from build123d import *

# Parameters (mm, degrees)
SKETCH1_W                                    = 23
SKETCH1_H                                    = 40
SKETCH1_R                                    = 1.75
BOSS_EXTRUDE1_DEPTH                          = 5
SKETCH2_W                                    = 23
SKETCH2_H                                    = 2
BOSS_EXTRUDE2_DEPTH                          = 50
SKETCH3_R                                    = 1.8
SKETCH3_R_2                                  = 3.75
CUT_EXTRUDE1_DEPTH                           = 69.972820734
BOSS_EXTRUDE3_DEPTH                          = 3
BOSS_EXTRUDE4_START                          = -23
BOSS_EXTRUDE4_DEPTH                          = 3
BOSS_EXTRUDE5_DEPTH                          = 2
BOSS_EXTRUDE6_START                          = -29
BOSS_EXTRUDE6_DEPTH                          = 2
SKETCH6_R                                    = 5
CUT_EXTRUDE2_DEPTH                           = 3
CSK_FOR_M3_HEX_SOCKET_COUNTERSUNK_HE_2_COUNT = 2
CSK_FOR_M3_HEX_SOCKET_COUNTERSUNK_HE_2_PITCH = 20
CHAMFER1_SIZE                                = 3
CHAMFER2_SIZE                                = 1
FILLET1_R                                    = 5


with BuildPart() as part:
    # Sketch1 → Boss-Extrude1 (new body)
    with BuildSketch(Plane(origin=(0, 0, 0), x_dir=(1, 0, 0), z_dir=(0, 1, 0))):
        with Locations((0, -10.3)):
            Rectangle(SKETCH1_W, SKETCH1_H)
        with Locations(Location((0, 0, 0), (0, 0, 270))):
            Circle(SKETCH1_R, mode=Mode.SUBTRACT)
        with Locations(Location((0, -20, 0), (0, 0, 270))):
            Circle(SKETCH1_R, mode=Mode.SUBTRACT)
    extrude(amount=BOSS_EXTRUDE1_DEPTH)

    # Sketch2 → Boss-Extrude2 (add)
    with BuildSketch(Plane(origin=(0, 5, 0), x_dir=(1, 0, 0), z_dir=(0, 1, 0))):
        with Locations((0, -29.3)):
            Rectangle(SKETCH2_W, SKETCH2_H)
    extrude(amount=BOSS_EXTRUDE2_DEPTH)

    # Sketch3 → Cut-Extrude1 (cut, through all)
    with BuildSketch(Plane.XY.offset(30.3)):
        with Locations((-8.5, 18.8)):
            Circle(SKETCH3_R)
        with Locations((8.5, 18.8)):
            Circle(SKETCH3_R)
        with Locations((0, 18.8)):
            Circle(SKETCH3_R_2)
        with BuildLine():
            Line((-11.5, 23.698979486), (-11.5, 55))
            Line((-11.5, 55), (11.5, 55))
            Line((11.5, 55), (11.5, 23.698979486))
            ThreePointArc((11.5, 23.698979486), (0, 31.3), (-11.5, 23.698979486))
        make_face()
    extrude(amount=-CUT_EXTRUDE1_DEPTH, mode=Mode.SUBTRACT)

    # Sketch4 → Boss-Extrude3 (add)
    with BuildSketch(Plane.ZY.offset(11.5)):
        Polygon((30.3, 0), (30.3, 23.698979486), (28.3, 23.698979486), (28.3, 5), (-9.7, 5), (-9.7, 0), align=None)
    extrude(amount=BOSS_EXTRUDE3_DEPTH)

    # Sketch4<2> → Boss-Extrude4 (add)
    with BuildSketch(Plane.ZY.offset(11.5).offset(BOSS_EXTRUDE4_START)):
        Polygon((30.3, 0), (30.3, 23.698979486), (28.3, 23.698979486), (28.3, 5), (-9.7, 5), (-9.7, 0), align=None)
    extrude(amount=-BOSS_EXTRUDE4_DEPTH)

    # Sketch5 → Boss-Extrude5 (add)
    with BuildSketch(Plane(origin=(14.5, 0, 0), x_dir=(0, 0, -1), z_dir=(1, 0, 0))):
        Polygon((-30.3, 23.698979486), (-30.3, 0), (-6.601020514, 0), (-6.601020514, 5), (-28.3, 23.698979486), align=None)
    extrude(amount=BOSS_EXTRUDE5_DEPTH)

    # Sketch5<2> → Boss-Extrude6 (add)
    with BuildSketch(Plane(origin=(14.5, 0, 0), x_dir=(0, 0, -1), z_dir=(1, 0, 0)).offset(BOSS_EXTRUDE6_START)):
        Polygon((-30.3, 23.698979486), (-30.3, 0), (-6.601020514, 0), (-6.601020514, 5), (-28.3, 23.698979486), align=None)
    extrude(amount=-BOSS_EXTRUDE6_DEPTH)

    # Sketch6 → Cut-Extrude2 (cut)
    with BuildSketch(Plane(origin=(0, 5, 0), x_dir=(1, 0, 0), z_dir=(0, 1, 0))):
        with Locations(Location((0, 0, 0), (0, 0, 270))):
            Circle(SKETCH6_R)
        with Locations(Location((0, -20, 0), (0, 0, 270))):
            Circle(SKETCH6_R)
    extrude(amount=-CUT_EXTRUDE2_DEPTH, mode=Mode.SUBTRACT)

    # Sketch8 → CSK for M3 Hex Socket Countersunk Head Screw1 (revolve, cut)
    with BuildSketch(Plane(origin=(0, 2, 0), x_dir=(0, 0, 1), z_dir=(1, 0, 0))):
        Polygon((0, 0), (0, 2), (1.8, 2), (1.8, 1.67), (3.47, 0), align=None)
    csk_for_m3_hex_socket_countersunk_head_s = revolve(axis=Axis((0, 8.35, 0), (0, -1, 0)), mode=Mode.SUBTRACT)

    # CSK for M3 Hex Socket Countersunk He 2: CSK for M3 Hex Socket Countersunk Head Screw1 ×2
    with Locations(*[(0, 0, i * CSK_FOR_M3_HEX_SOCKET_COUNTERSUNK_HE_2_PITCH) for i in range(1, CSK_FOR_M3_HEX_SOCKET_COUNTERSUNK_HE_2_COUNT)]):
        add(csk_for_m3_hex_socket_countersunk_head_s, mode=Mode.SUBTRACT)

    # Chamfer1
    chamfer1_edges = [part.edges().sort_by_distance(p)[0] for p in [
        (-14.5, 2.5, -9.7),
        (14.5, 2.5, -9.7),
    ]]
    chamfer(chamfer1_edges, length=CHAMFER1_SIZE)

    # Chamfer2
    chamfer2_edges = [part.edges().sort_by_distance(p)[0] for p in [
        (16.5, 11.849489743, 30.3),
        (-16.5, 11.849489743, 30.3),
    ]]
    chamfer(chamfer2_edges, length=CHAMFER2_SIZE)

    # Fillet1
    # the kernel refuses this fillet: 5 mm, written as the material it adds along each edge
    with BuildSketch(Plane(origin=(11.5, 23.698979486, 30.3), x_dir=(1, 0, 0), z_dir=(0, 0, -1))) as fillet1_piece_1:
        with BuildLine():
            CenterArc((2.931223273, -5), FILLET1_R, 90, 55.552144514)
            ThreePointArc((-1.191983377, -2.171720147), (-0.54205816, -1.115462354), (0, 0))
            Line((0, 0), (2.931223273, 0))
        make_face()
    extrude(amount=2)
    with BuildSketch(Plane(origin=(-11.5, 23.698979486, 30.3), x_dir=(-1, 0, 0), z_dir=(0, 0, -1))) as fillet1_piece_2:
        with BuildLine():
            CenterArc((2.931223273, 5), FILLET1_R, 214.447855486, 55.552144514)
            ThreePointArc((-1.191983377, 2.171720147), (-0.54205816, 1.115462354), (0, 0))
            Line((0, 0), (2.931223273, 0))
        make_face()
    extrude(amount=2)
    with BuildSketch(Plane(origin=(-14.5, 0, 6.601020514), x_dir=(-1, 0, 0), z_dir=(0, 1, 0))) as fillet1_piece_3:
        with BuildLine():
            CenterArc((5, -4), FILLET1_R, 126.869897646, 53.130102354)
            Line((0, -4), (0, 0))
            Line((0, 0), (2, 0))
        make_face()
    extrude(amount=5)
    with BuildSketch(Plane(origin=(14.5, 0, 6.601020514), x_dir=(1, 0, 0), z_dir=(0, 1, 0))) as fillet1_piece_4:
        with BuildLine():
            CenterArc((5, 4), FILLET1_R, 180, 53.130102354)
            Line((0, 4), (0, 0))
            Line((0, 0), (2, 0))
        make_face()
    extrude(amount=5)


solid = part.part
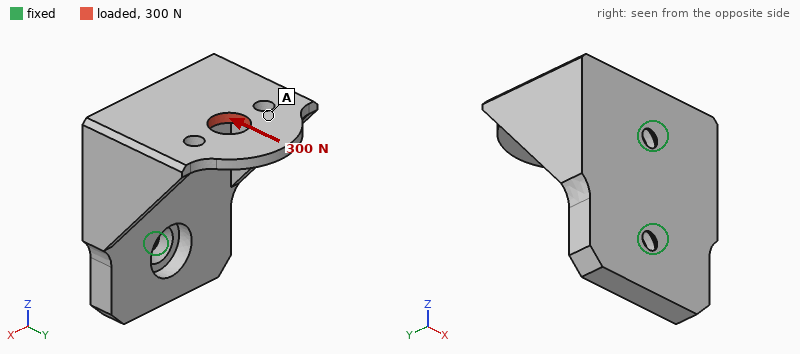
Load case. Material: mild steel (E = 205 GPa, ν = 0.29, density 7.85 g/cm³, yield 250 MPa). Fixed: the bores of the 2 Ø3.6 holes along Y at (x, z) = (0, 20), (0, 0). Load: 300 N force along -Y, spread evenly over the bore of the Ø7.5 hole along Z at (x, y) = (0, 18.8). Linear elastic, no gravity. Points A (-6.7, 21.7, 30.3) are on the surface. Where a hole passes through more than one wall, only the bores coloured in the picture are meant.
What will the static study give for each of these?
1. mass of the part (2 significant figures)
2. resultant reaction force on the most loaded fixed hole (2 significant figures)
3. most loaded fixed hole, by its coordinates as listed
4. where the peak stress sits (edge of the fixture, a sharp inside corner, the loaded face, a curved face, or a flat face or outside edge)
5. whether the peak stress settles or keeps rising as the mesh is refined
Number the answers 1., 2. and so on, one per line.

1. 62 g
2. 450 N
3. (0, 20)
4. edge of the fixture
5. keeps rising
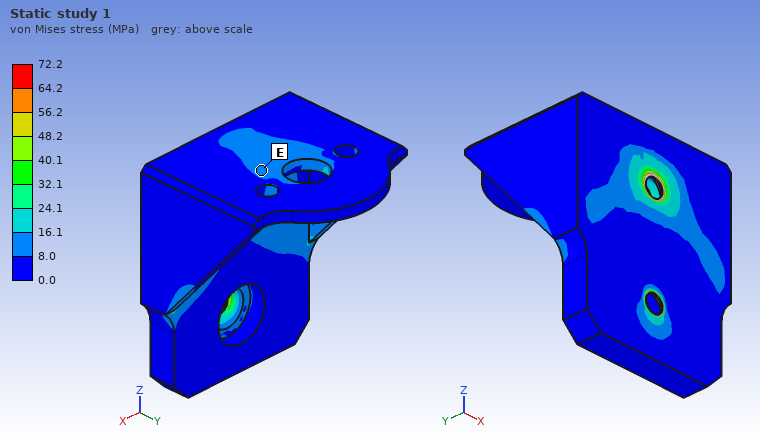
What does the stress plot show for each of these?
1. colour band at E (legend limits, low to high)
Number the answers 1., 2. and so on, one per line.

1. 8.0 to 16.1 MPa
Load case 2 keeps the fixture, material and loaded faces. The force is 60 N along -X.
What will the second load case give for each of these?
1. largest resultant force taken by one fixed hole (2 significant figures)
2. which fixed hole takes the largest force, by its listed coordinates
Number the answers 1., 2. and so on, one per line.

1. 82 N
2. (0, 20)
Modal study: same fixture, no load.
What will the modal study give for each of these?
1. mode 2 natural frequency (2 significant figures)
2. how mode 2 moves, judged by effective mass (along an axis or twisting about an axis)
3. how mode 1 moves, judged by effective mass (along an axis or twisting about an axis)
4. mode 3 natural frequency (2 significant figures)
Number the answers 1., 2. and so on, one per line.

1. 4800 Hz
2. along Z
3. along X
4. 7300 Hz
